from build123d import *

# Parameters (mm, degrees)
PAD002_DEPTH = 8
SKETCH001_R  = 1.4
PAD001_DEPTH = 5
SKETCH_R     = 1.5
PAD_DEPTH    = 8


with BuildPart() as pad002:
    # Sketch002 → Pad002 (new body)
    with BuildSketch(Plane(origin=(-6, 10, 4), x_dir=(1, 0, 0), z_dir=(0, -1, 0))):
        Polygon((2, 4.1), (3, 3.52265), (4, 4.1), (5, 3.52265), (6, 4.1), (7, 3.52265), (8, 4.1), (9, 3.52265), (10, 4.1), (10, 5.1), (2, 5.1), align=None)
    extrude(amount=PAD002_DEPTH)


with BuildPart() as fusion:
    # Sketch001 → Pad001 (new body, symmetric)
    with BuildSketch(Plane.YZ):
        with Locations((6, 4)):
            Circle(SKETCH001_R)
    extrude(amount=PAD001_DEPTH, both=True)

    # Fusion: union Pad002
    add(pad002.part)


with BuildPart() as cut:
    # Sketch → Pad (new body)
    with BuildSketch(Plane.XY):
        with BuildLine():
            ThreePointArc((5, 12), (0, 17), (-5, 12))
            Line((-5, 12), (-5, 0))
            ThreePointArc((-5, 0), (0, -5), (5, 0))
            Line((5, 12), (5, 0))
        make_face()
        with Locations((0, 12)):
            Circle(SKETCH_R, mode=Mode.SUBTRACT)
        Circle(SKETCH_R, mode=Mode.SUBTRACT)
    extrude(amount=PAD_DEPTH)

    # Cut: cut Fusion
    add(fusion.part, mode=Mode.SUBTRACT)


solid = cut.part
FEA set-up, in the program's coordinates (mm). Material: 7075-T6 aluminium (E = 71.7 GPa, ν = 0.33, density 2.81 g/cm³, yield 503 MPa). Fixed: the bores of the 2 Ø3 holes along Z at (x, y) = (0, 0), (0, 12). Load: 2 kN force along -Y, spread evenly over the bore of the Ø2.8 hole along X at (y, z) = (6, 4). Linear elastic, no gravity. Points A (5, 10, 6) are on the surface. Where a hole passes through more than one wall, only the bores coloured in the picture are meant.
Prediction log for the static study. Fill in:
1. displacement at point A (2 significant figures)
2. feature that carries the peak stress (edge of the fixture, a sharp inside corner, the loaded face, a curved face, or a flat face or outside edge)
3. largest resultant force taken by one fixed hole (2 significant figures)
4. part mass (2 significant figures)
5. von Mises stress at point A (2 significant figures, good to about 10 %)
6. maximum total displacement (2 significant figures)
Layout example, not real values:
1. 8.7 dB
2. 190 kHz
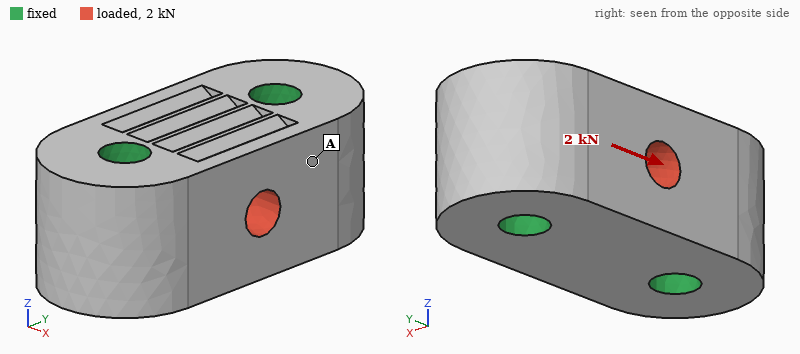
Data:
1. 0.85 µm
2. the loaded face
3. 1.0 kN
4. 3.9 g
5. 8.7 MPa
6. 1.6 µm
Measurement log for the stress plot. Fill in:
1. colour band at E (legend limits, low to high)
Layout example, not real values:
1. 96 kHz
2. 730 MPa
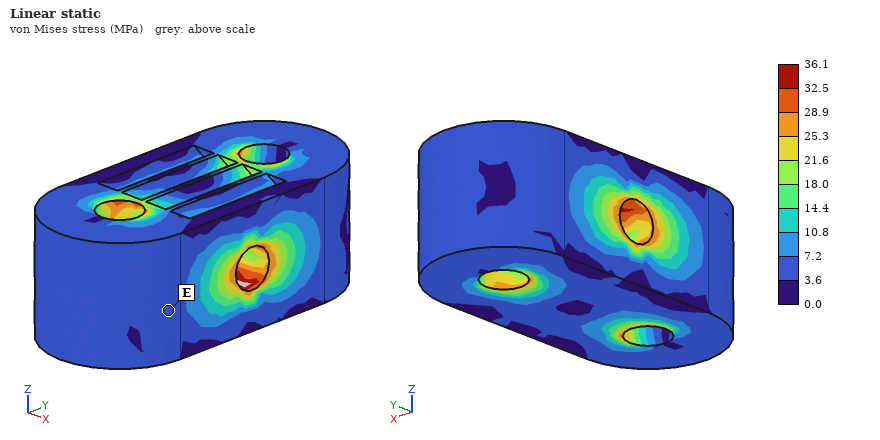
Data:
1. 3.6 to 7.2 MPa
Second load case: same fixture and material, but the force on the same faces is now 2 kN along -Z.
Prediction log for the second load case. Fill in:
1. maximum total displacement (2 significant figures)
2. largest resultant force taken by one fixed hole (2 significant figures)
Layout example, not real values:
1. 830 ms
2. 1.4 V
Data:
1. 3.9 µm
2. 1.0 kN
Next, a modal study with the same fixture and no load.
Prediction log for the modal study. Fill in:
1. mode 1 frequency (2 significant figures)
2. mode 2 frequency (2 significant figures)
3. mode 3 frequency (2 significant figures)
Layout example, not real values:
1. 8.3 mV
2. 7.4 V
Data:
1. 110 kHz
2. 110 kHz
3. 120 kHz
